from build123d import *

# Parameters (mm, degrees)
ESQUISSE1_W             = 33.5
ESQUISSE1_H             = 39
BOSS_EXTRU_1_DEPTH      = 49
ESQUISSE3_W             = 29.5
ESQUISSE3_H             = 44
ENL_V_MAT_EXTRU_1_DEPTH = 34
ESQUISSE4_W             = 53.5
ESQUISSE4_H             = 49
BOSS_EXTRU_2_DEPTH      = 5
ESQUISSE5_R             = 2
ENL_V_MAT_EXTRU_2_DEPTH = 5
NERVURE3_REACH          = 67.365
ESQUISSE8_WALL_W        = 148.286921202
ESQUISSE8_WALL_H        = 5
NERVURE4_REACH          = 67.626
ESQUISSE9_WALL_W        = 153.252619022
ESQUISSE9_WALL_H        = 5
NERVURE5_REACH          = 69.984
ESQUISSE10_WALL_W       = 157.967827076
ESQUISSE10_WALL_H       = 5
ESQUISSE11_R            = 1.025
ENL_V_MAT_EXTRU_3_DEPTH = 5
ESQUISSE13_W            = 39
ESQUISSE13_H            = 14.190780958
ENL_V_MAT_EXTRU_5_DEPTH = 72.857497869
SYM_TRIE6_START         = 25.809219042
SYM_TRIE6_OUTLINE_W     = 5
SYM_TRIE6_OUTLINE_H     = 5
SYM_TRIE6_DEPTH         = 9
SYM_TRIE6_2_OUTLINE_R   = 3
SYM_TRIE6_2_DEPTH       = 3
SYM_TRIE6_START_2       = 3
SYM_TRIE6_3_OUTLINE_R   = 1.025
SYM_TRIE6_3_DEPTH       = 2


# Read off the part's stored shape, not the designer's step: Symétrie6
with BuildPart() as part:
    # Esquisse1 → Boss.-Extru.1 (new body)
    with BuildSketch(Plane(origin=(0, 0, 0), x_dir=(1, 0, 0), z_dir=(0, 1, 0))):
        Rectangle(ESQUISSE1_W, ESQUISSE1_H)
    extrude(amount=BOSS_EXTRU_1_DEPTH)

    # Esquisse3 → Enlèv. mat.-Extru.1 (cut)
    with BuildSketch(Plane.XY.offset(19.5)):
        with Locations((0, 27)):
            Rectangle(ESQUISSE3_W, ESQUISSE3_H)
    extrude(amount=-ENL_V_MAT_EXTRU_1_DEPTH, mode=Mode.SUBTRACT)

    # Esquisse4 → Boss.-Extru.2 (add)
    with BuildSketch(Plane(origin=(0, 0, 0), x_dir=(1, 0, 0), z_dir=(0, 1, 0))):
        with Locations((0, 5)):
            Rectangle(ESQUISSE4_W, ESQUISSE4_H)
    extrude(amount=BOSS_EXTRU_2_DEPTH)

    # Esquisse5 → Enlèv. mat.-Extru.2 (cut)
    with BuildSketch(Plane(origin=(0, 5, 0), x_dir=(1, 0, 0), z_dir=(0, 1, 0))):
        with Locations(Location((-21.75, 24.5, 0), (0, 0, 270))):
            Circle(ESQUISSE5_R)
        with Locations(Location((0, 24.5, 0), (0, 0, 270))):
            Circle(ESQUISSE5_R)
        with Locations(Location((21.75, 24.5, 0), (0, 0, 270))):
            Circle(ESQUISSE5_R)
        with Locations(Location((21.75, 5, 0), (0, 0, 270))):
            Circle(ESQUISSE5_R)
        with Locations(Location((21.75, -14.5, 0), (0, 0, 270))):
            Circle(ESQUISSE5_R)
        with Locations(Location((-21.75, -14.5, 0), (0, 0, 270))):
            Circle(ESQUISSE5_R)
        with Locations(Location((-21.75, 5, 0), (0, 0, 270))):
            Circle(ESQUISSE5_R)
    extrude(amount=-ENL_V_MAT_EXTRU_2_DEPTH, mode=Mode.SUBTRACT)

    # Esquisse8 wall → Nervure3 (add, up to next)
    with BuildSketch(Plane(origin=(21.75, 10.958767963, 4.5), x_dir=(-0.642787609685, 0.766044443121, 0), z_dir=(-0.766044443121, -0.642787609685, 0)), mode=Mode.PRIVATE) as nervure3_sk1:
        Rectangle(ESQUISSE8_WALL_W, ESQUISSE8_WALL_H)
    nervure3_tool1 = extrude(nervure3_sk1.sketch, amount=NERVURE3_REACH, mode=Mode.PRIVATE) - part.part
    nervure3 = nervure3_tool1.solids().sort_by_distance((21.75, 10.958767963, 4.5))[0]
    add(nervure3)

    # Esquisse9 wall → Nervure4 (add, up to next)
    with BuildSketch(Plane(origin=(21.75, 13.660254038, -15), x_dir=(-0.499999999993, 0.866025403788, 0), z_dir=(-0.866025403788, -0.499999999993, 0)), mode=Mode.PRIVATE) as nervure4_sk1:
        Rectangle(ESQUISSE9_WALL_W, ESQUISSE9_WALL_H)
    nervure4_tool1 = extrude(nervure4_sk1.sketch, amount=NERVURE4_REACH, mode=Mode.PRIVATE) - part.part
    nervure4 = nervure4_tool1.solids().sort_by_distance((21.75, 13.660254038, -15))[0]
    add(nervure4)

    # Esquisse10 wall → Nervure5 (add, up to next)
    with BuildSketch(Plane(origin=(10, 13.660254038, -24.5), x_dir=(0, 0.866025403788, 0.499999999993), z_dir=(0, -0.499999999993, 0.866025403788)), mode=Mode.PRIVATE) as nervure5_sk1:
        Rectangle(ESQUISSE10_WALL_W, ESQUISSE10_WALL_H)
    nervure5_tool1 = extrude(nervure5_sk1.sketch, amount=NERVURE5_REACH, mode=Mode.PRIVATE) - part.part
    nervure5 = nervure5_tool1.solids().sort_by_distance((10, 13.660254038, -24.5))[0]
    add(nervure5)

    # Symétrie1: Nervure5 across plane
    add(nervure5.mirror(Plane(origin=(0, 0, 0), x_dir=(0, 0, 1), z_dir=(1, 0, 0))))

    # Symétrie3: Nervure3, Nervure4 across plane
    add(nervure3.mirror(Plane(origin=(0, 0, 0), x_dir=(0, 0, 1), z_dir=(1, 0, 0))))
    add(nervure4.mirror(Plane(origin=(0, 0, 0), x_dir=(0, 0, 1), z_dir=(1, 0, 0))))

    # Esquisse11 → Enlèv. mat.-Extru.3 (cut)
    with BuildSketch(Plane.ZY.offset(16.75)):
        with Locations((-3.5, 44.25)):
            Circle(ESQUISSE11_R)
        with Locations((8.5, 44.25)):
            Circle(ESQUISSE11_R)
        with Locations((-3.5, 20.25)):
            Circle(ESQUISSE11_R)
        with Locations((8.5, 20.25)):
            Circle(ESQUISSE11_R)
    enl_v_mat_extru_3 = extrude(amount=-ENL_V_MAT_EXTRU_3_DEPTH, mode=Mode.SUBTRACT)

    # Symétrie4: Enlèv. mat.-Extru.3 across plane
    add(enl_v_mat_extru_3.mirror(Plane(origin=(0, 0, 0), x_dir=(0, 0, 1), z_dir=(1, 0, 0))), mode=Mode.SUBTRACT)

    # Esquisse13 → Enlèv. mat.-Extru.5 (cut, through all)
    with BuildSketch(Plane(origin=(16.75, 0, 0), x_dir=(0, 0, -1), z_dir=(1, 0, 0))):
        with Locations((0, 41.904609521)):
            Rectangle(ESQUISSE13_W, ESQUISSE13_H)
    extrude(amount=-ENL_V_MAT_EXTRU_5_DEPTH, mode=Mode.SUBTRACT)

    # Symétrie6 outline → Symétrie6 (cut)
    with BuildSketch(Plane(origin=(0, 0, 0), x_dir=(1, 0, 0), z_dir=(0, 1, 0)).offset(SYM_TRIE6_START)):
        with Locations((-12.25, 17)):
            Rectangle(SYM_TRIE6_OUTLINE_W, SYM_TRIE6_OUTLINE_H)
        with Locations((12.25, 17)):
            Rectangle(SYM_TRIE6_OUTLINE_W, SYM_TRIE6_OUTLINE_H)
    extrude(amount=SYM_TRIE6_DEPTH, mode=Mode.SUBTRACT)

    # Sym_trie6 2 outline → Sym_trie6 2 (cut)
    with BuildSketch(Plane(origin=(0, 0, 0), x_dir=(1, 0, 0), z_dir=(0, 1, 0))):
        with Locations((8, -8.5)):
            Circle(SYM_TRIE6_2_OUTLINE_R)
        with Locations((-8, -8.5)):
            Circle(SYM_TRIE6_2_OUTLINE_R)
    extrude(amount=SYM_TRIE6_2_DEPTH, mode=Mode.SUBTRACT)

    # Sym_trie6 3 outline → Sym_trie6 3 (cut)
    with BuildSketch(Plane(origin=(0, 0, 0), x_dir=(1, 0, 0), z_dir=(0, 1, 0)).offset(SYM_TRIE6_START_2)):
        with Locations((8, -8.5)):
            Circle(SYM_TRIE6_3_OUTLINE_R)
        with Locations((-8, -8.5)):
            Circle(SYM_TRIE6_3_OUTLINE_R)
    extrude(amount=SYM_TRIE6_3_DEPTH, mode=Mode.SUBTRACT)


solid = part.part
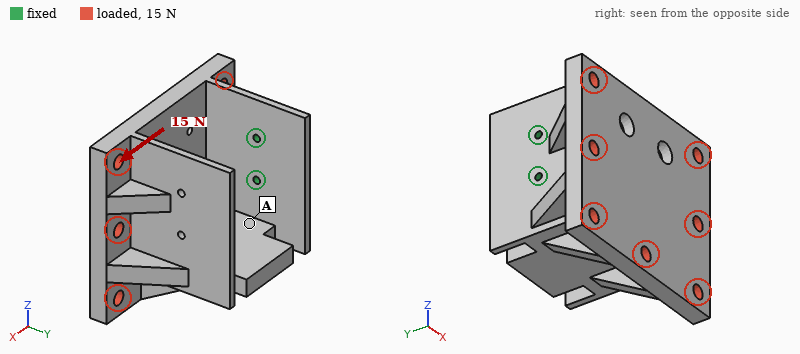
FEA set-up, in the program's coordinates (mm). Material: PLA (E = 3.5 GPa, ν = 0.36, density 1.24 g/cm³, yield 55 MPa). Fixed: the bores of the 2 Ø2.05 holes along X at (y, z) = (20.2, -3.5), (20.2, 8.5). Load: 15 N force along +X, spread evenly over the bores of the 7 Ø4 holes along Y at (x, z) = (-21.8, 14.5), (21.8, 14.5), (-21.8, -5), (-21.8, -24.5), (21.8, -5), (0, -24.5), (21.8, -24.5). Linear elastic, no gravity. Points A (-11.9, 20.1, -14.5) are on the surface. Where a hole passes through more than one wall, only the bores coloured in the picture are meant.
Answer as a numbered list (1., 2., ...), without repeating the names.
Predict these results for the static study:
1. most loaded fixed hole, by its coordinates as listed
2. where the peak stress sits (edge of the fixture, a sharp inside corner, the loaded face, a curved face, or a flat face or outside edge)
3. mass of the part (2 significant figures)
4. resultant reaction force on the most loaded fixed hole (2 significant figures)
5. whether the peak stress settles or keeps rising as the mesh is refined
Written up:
1. (20.2, -3.5)
2. edge of the fixture
3. 29 g
4. 18 N
5. keeps rising
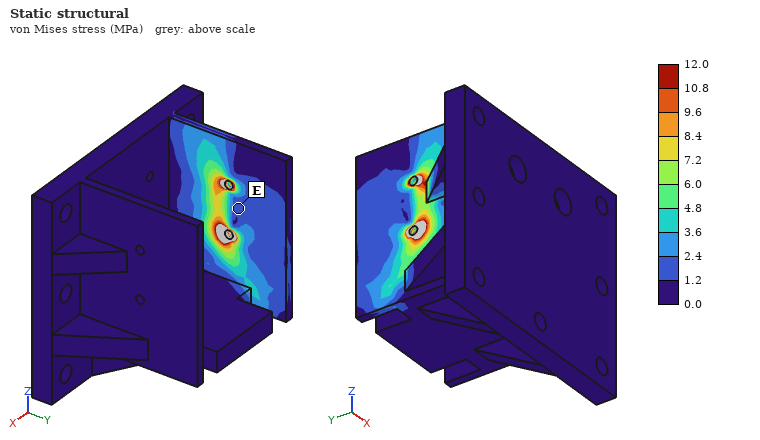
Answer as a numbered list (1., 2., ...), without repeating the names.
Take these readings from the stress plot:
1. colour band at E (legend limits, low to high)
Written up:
1. 1.2 to 2.4 MPa
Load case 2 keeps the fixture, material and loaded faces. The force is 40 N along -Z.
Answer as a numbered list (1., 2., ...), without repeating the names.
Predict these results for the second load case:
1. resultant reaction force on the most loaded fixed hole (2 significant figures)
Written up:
1. 71 N
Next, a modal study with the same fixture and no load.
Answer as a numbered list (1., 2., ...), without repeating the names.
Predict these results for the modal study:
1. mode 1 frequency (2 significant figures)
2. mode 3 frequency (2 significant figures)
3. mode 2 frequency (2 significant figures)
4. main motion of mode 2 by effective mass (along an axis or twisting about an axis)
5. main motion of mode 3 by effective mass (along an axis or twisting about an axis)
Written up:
1. 140 Hz
2. 810 Hz
3. 260 Hz
4. along Z
5. along X
